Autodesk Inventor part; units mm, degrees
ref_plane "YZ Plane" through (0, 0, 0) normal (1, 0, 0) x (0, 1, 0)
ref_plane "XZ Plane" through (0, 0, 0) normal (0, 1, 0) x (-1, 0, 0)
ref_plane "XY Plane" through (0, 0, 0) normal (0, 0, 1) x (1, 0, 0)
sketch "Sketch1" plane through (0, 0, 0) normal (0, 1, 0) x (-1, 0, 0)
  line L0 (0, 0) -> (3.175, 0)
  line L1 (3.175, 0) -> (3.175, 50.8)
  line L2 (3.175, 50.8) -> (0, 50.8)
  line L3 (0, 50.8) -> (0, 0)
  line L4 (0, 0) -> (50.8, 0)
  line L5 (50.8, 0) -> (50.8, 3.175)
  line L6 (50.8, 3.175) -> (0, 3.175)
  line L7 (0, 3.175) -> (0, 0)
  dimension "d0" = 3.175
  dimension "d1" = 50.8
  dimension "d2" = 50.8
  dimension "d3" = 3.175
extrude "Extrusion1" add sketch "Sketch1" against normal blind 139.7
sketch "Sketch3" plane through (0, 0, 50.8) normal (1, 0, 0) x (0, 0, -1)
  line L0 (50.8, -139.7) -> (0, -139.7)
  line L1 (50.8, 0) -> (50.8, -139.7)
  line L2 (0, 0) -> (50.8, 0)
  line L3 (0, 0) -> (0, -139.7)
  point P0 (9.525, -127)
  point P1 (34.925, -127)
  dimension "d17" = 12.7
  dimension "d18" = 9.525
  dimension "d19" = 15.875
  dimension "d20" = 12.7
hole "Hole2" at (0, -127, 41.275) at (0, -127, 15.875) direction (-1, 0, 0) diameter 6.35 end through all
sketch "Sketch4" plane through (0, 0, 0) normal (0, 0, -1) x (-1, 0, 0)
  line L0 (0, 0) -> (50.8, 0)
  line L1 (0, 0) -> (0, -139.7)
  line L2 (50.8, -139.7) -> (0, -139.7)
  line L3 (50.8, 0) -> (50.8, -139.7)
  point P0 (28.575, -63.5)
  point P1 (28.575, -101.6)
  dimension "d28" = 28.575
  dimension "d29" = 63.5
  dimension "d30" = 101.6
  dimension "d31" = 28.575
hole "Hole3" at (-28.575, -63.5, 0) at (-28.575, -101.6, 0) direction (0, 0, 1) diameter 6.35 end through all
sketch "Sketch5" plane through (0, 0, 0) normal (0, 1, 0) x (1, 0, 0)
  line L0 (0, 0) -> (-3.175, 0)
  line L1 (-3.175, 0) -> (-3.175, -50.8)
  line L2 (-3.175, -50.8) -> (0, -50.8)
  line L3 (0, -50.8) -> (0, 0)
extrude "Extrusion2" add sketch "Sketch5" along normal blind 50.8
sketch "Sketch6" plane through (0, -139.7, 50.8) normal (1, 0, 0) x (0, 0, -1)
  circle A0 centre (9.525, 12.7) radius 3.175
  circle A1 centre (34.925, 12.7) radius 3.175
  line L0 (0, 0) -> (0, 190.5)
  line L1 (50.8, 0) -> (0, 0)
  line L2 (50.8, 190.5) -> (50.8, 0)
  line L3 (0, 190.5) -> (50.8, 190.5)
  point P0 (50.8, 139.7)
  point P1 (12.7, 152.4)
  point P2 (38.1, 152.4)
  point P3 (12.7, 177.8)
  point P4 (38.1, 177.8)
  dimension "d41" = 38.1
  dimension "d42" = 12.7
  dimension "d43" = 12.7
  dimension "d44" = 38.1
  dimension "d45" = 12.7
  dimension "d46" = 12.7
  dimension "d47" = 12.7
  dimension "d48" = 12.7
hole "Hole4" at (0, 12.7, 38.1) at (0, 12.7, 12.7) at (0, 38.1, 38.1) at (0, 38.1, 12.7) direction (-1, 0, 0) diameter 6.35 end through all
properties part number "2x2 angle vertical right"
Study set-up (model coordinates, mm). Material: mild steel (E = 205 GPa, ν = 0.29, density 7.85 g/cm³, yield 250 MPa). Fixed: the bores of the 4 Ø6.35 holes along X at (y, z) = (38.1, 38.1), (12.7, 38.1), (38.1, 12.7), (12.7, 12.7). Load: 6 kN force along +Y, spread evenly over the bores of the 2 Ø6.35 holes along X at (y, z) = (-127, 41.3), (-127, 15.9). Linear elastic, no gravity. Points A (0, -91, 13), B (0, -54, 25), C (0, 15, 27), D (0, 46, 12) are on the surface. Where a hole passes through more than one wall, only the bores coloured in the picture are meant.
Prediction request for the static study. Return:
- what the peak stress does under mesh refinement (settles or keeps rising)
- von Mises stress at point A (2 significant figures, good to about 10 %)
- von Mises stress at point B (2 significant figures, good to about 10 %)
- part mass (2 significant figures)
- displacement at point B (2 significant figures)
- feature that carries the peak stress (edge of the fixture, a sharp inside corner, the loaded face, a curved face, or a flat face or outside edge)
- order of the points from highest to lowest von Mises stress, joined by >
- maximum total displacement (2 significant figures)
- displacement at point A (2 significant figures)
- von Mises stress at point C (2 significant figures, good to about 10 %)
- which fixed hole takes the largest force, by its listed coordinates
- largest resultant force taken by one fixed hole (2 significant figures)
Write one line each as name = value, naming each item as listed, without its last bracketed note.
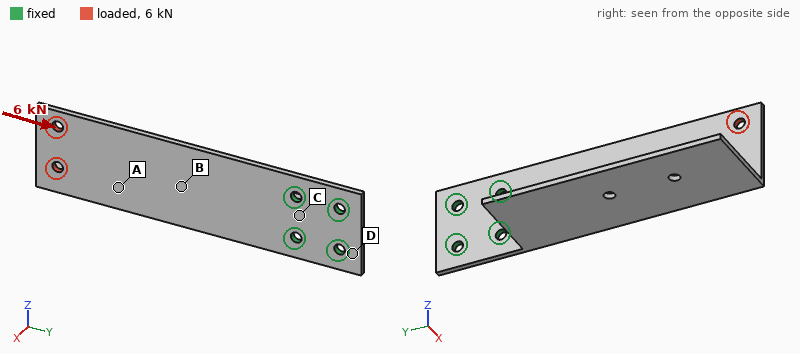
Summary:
what the peak stress does under mesh refinement = keeps rising
von Mises stress at point A = 26 MPa
von Mises stress at point B = 35 MPa
part mass = 400 g
displacement at point B = 15 µm
feature that carries the peak stress = edge of the fixture
order of the points from highest to lowest von Mises stress, joined by > = B > A > C > D
maximum total displacement = 63 µm
displacement at point A = 27 µm
von Mises stress at point C = 16 MPa
which fixed hole takes the largest force, by its listed coordinates = (12.7, 38.1)
largest resultant force taken by one fixed hole = 3.1 kN
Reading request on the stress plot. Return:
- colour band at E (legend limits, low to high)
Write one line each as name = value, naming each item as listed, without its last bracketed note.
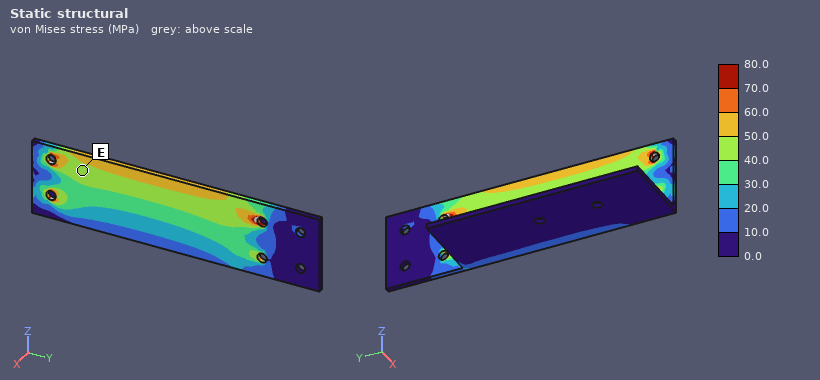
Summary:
colour band at E = 40.0 to 50.0 MPa
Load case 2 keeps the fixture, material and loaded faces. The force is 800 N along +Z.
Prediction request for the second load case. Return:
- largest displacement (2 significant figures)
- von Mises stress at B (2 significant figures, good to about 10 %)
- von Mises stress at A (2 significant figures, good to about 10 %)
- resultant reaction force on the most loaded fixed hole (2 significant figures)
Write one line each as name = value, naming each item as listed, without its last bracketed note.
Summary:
largest displacement = 0.13 mm
von Mises stress at B = 12 MPa
von Mises stress at A = 12 MPa
resultant reaction force on the most loaded fixed hole = 3.0 kN
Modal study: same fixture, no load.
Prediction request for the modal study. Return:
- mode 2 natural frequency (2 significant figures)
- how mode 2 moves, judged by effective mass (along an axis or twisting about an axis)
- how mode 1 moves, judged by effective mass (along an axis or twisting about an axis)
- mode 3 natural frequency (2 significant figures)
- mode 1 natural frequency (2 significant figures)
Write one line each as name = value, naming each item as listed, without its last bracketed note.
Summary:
mode 2 natural frequency = 340 Hz
how mode 2 moves, judged by effective mass = along Z
how mode 1 moves, judged by effective mass = along X
mode 3 natural frequency = 1000 Hz
mode 1 natural frequency = 110 Hz
